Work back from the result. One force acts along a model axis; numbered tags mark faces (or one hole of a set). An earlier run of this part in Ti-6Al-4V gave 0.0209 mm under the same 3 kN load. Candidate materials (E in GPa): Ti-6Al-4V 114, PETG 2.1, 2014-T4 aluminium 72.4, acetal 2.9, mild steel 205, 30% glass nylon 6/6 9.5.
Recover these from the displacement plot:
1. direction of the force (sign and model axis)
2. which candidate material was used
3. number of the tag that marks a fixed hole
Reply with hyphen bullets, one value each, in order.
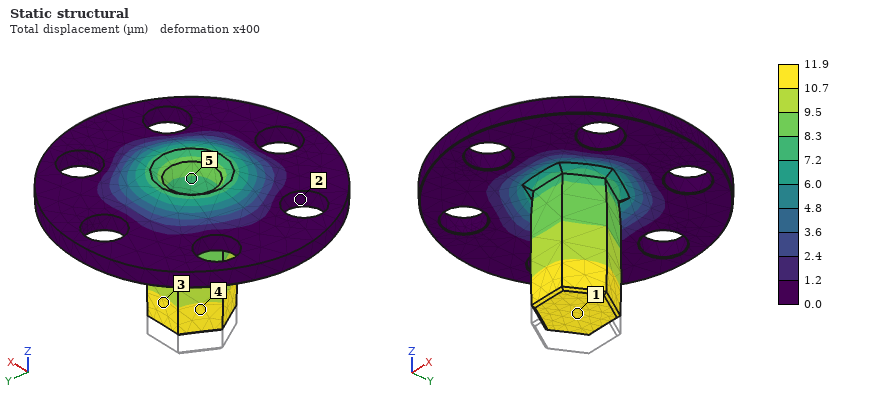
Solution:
- +Z
- mild steel
- 2
